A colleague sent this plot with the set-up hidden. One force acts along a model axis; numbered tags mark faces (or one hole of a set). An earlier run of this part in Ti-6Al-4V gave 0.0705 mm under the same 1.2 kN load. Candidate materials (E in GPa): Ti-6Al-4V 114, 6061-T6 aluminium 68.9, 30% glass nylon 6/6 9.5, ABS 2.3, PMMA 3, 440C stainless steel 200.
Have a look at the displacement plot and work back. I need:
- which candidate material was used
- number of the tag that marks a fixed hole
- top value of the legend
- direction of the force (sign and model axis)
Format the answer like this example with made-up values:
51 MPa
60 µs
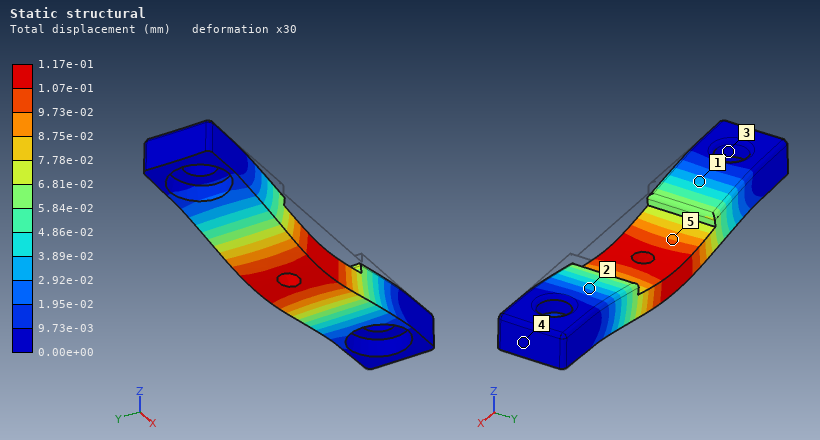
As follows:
6061-T6 aluminium
3
1.17e-01 mm
-Z
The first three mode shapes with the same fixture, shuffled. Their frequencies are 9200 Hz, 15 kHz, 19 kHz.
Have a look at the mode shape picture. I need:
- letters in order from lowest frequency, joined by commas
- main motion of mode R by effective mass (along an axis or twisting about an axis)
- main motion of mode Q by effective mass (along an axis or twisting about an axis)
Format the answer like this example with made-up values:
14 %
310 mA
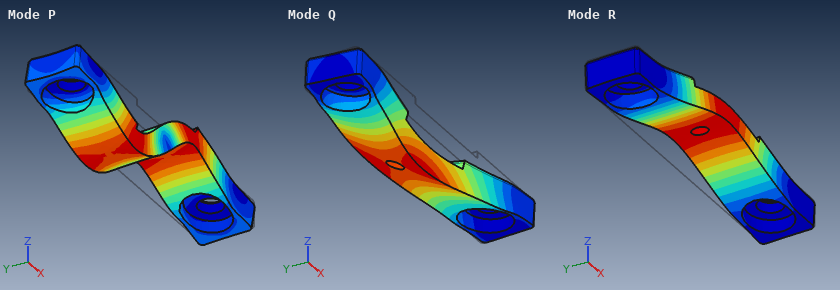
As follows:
R, Q, P
along Z
along Y
